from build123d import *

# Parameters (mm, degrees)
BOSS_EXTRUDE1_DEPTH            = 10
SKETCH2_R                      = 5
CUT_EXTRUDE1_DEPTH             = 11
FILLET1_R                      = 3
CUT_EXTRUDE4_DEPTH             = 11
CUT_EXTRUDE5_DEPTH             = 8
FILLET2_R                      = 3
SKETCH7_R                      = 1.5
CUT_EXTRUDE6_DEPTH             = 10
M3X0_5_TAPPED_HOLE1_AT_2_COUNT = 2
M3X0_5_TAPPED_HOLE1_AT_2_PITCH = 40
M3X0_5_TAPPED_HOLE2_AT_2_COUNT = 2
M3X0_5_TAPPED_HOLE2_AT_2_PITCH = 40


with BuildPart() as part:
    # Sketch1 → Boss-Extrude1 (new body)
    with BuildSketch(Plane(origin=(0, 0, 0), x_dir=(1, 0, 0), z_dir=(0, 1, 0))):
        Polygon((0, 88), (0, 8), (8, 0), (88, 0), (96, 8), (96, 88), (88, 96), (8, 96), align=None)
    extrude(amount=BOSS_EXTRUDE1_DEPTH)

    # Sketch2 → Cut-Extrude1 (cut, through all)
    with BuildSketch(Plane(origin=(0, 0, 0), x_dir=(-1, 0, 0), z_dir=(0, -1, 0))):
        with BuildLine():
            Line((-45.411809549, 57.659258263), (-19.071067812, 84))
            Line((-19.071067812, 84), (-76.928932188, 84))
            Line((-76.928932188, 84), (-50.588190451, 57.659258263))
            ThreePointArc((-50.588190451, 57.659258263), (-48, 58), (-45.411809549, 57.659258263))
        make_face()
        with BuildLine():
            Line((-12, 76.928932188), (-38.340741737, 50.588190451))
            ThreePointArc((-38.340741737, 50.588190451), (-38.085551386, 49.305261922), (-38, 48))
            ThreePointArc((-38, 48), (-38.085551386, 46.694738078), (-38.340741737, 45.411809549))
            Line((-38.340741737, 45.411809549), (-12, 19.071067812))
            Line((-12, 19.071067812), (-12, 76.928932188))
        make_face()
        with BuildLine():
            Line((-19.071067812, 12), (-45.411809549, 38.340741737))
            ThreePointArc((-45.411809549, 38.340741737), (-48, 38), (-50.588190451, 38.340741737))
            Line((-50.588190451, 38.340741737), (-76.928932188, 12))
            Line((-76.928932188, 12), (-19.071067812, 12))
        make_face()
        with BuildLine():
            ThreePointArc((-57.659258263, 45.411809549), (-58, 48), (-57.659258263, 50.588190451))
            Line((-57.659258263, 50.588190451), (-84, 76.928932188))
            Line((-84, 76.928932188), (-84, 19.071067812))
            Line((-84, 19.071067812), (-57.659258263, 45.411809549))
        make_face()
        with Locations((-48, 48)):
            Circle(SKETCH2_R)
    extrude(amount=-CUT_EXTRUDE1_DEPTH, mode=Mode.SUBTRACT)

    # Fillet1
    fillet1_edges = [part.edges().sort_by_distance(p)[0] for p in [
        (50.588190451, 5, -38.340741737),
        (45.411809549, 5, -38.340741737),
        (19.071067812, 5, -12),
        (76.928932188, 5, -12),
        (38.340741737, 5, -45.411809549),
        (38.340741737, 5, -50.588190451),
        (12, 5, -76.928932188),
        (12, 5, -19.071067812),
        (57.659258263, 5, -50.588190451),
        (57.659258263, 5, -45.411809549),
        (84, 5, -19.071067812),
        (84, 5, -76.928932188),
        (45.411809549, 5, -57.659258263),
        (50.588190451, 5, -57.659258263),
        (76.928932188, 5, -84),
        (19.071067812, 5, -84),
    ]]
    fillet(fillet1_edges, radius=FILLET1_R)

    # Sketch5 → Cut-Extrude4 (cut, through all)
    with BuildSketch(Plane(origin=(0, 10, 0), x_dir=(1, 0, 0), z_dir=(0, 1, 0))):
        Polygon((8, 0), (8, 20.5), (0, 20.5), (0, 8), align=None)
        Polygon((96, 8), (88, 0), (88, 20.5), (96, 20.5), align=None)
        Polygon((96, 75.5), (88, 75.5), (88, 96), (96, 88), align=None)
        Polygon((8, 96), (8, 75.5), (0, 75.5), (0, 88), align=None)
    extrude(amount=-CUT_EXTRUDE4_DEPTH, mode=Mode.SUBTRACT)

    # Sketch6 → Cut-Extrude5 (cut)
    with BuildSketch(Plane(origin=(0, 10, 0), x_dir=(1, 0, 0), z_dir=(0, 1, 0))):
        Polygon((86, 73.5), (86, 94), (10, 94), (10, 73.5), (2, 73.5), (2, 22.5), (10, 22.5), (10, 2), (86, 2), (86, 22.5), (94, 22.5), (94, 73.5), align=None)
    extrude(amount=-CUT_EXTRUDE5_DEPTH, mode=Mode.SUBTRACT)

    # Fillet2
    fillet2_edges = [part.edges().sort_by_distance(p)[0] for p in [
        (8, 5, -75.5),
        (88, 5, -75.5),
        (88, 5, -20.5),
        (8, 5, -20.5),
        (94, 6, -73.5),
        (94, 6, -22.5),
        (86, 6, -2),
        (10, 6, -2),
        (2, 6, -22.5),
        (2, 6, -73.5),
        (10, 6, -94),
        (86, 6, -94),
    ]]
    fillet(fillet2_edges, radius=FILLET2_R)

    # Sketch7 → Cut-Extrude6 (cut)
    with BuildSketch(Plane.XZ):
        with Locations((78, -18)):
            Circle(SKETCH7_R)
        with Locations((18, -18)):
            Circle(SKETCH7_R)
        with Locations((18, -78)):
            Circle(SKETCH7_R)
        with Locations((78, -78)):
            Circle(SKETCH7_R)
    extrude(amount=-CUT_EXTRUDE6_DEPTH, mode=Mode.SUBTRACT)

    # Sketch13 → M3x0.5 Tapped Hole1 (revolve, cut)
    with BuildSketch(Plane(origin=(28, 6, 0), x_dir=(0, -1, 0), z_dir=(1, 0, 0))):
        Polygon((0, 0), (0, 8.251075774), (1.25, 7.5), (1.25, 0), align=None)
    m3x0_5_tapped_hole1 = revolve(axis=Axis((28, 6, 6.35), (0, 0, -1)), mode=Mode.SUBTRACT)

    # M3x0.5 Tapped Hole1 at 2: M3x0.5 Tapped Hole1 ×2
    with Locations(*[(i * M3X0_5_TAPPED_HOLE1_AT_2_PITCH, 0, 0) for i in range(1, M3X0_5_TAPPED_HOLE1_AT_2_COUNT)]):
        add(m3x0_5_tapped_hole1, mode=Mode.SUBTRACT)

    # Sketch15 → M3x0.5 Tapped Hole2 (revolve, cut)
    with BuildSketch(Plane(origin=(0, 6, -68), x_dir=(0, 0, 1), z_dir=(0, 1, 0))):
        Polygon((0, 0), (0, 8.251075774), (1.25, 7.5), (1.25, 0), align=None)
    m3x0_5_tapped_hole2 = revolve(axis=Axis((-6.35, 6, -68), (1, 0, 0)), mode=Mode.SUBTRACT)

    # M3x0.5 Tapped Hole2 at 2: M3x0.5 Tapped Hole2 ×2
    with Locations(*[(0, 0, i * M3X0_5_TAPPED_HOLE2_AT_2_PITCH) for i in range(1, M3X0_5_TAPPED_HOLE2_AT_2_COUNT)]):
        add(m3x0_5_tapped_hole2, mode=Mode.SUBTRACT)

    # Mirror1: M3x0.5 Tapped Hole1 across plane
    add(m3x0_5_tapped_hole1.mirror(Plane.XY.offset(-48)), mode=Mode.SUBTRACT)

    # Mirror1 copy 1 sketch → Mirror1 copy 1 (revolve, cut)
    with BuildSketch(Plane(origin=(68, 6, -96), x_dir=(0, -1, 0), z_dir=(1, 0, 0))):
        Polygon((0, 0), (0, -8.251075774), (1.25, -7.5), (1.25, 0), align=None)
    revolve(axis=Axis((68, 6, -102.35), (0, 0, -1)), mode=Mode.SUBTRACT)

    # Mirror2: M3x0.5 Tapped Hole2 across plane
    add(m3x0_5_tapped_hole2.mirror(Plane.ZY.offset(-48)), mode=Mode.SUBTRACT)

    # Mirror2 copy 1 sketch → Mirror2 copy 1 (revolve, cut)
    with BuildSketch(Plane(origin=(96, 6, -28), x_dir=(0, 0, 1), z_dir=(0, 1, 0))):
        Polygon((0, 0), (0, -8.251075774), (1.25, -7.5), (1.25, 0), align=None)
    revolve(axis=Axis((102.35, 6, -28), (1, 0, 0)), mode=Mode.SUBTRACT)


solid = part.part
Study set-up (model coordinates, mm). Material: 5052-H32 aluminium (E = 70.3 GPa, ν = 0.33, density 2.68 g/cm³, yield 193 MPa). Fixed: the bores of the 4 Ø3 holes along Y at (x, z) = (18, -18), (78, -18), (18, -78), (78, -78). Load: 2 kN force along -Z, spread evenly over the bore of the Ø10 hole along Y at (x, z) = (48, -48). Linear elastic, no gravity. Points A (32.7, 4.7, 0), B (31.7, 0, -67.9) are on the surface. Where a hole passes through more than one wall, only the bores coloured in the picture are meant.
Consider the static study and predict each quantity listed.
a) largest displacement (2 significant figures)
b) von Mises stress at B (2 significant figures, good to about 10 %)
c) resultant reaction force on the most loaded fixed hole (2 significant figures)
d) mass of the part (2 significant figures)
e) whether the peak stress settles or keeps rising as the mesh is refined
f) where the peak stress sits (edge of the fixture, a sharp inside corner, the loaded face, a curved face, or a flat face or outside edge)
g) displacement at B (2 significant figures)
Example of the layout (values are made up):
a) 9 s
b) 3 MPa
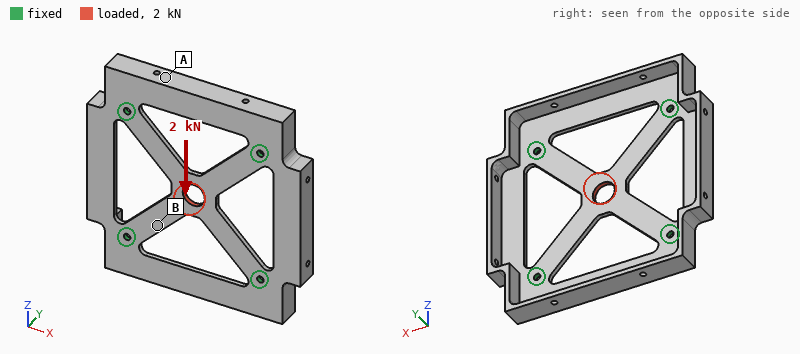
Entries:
a) 29 µm
b) 36 MPa
c) 650 N
d) 44 g
e) keeps rising
f) edge of the fixture
g) 12 µm
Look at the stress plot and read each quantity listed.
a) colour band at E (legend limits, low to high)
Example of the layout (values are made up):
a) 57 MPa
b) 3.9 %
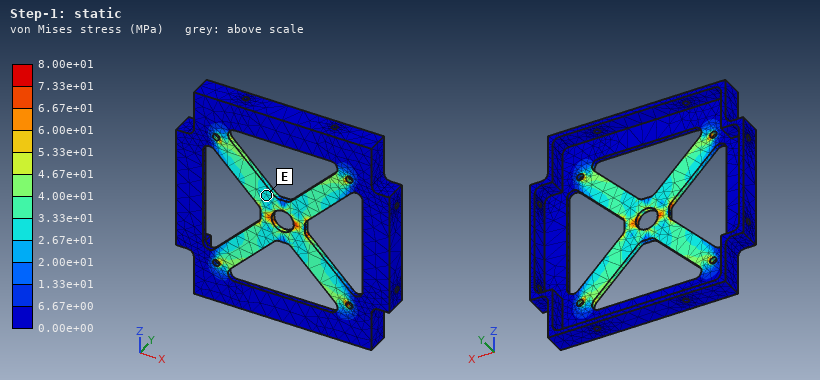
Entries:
a) 2.67e+01 to 3.33e+01 MPa
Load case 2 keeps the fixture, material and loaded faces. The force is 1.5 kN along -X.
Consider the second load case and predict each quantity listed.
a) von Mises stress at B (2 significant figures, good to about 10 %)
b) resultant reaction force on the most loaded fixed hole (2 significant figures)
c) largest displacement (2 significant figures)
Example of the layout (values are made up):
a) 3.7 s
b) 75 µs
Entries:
a) 24 MPa
b) 490 N
c) 22 µm
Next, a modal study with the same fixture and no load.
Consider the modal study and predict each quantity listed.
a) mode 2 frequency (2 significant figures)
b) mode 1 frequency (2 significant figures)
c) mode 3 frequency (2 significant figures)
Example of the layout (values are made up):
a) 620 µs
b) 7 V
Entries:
a) 2300 Hz
b) 1800 Hz
c) 2600 Hz
